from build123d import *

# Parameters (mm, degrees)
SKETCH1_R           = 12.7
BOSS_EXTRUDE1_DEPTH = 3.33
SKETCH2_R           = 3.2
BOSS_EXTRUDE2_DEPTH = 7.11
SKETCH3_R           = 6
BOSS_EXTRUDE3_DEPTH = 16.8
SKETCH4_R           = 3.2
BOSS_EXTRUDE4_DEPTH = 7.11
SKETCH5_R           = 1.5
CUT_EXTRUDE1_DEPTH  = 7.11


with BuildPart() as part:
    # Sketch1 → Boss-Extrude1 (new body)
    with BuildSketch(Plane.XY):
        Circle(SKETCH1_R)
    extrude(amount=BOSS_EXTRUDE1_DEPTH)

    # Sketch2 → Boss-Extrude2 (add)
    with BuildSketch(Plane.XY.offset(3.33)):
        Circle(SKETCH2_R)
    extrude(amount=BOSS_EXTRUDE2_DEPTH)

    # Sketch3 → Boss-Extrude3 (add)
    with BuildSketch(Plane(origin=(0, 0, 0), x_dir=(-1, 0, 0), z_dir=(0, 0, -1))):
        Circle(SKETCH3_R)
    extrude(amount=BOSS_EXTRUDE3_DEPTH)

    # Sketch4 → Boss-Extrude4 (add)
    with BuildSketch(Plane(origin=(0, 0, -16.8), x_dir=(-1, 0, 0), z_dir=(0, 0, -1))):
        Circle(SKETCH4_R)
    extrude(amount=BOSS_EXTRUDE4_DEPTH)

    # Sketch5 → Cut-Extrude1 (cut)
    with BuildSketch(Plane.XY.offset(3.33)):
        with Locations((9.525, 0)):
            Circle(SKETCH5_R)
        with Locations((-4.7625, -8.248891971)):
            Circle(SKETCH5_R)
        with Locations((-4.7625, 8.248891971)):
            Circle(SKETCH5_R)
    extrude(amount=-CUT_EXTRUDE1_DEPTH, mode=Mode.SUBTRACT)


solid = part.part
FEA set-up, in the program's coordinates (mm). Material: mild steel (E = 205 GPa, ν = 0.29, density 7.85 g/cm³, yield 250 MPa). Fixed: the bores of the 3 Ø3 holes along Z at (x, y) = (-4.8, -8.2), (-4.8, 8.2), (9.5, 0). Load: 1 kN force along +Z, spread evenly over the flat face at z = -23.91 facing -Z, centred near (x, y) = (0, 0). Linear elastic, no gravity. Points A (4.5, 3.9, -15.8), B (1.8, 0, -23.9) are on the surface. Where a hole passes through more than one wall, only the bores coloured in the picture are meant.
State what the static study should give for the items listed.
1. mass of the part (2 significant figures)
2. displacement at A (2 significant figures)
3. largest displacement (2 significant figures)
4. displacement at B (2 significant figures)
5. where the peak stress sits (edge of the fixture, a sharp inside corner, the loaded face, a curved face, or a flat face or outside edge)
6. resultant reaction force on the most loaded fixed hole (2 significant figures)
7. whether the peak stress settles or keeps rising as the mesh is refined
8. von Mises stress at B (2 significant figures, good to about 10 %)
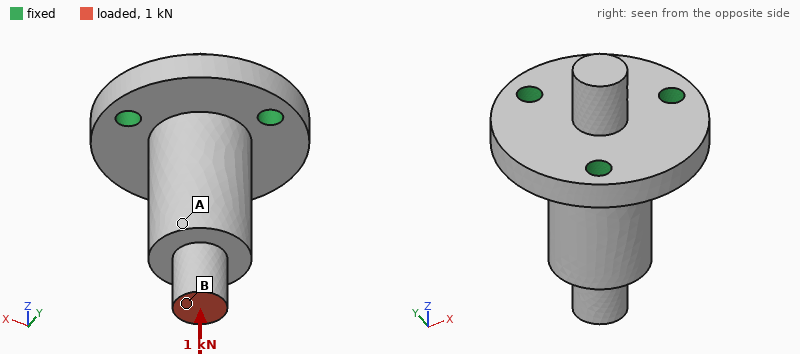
31 g
1.7 µm
3.1 µm
3.1 µm
edge of the fixture
340 N
keeps rising
31 MPa
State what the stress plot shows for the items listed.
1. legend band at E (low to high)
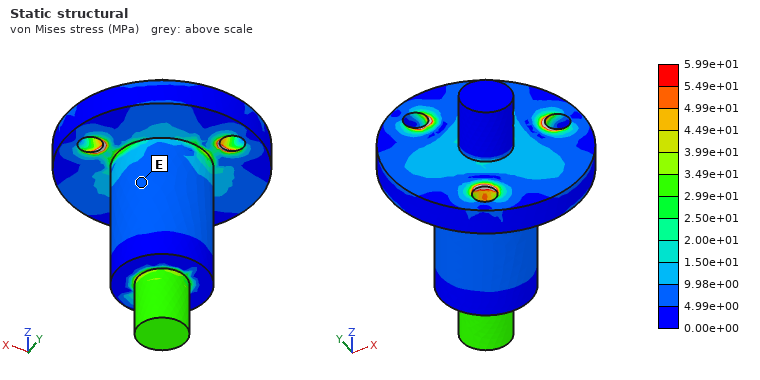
4.99e+00 to 9.98e+00 MPa
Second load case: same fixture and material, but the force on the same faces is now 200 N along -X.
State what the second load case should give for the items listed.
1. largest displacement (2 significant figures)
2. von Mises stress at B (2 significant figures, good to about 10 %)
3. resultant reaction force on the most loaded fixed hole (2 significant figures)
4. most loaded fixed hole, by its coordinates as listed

12 µm
15 MPa
390 N
(9.5, 0)
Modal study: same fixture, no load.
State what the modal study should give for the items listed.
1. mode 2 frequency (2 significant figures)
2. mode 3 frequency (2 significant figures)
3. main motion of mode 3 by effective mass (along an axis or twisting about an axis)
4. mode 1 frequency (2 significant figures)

12 kHz
29 kHz
along Z
12 kHz
